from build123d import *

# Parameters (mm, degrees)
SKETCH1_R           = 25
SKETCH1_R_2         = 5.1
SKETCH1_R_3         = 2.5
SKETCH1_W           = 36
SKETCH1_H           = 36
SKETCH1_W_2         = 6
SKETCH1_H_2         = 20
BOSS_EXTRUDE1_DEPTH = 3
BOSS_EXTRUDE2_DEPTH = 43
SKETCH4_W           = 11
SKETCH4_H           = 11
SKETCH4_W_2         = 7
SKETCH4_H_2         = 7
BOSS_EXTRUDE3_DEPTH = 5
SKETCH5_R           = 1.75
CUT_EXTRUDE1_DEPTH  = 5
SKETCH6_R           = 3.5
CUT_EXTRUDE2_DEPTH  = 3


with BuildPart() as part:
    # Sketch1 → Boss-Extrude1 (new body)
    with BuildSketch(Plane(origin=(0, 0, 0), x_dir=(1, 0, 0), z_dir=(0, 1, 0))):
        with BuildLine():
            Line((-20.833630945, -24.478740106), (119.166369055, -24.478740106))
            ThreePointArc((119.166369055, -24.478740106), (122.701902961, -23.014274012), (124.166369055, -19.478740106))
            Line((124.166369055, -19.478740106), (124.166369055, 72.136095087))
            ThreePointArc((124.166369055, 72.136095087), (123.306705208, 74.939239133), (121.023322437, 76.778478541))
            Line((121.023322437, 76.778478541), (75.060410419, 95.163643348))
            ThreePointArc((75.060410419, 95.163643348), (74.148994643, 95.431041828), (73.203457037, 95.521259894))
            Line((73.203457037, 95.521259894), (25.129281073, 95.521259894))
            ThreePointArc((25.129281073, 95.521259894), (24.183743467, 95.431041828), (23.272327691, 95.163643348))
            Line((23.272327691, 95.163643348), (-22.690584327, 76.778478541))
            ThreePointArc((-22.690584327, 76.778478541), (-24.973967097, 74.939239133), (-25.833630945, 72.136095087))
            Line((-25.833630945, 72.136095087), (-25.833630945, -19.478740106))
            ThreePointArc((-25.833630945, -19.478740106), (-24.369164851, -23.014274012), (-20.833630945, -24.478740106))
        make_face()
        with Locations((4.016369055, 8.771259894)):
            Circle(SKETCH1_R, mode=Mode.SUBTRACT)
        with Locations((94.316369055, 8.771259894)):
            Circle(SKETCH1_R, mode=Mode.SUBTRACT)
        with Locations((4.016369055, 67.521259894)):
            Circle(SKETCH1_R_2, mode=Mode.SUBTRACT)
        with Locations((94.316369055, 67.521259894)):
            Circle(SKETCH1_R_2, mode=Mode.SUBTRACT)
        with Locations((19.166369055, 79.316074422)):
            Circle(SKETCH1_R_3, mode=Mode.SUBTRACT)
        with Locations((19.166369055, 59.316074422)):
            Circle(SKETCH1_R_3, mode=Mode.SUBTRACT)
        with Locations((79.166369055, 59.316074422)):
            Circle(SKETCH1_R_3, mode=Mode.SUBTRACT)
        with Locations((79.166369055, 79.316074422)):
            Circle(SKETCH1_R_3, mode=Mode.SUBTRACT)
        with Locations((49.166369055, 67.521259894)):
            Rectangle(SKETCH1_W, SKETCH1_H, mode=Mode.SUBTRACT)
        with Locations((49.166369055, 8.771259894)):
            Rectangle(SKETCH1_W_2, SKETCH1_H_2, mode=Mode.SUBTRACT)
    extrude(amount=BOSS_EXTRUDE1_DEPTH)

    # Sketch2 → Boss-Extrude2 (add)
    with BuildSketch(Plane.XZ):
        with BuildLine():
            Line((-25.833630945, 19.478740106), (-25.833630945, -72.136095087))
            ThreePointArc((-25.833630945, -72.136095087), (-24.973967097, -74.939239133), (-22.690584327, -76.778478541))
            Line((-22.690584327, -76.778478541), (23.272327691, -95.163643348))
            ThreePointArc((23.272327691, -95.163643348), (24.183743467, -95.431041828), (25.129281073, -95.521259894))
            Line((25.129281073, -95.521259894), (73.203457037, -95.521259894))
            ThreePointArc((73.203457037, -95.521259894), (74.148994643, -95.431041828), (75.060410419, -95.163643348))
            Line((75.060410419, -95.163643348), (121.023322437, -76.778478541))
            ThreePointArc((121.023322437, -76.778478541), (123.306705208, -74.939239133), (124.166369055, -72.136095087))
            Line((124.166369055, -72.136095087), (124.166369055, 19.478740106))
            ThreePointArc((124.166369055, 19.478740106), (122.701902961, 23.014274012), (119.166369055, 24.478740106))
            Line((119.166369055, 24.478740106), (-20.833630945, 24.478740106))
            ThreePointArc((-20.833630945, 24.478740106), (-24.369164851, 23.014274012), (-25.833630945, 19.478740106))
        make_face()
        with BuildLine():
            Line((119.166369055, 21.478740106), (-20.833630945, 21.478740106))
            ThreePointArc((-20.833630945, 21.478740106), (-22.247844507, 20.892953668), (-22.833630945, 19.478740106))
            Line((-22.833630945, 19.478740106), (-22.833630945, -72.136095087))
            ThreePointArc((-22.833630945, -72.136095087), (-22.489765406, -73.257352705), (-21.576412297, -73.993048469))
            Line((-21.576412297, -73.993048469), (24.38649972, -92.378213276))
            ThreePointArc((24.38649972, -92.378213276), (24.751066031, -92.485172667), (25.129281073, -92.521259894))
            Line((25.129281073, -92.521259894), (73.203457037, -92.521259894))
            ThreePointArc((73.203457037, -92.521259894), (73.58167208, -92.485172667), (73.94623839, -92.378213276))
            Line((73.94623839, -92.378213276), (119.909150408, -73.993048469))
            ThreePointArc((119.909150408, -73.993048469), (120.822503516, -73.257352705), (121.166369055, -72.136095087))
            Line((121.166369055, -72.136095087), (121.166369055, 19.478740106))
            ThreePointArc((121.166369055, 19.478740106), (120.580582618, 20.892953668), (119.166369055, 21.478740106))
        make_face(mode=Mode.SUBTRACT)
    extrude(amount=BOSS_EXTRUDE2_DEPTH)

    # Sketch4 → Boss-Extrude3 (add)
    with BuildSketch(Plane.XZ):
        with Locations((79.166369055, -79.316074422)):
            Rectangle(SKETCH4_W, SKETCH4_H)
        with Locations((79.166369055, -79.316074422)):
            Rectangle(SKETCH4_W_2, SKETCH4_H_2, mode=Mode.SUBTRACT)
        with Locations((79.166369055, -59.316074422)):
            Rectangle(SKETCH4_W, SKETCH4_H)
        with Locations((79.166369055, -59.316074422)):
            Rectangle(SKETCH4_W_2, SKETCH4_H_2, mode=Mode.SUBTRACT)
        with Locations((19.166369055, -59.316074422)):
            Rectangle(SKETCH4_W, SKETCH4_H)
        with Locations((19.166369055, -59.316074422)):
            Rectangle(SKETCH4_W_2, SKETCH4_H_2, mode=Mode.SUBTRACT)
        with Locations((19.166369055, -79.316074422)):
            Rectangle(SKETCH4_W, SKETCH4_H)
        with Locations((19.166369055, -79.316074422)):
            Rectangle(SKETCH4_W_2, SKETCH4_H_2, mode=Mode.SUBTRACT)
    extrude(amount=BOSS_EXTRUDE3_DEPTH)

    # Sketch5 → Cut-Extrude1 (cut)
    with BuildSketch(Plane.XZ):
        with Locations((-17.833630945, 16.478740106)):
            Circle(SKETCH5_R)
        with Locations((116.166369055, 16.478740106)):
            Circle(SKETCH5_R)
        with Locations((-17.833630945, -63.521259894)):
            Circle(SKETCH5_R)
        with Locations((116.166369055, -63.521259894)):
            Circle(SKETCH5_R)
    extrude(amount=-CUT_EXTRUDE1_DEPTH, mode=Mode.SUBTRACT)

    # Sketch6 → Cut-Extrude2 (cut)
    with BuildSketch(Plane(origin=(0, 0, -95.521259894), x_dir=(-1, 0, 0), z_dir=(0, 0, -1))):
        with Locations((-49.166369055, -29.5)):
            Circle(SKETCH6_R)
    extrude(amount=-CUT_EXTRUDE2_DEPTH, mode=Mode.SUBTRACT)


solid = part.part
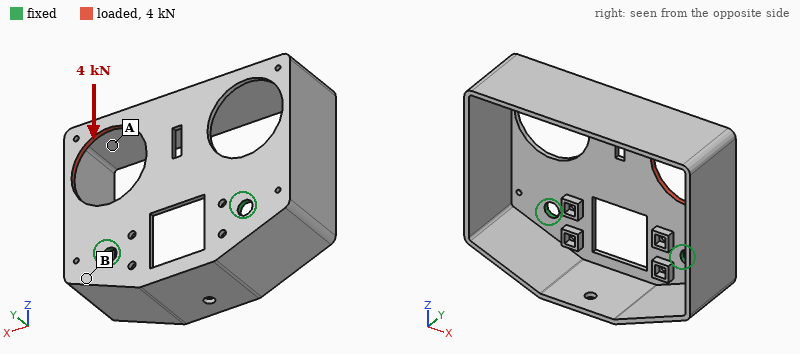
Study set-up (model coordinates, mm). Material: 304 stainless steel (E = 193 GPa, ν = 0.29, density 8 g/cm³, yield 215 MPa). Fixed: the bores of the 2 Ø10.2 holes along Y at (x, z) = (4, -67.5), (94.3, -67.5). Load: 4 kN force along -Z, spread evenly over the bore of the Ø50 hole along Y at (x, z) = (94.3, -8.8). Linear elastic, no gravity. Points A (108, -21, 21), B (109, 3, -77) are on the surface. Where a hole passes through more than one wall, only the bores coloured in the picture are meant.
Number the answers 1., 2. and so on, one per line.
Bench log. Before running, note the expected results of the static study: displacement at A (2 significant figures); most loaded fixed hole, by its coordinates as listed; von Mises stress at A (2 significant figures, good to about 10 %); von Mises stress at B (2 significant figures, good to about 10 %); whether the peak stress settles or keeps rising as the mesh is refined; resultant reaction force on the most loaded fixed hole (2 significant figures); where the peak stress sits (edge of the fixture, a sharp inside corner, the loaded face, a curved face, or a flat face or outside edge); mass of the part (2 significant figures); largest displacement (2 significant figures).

1. 26 µm
2. (94.3, -67.5)
3. 8.3 MPa
4. 21 MPa
5. keeps rising
6. 3.8 kN
7. edge of the fixture
8. 790 g
9. 36 µm
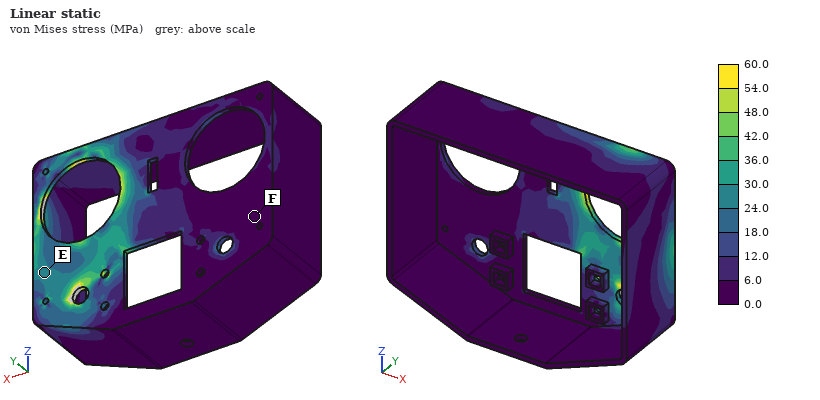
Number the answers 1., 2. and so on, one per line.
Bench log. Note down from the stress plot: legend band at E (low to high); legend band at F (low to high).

1. 24.0 to 30.0 MPa
2. 0.0 to 6.0 MPa
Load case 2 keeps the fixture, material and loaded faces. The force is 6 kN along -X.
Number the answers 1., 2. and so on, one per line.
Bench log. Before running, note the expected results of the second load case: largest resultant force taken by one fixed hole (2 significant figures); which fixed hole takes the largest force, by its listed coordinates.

1. 4.8 kN
2. (94.3, -67.5)
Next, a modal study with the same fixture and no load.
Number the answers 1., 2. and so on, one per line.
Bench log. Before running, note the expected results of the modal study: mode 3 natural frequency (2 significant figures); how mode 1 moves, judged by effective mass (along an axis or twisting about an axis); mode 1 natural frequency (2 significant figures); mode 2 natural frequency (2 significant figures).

1. 970 Hz
2. along Y
3. 260 Hz
4. 410 Hz
